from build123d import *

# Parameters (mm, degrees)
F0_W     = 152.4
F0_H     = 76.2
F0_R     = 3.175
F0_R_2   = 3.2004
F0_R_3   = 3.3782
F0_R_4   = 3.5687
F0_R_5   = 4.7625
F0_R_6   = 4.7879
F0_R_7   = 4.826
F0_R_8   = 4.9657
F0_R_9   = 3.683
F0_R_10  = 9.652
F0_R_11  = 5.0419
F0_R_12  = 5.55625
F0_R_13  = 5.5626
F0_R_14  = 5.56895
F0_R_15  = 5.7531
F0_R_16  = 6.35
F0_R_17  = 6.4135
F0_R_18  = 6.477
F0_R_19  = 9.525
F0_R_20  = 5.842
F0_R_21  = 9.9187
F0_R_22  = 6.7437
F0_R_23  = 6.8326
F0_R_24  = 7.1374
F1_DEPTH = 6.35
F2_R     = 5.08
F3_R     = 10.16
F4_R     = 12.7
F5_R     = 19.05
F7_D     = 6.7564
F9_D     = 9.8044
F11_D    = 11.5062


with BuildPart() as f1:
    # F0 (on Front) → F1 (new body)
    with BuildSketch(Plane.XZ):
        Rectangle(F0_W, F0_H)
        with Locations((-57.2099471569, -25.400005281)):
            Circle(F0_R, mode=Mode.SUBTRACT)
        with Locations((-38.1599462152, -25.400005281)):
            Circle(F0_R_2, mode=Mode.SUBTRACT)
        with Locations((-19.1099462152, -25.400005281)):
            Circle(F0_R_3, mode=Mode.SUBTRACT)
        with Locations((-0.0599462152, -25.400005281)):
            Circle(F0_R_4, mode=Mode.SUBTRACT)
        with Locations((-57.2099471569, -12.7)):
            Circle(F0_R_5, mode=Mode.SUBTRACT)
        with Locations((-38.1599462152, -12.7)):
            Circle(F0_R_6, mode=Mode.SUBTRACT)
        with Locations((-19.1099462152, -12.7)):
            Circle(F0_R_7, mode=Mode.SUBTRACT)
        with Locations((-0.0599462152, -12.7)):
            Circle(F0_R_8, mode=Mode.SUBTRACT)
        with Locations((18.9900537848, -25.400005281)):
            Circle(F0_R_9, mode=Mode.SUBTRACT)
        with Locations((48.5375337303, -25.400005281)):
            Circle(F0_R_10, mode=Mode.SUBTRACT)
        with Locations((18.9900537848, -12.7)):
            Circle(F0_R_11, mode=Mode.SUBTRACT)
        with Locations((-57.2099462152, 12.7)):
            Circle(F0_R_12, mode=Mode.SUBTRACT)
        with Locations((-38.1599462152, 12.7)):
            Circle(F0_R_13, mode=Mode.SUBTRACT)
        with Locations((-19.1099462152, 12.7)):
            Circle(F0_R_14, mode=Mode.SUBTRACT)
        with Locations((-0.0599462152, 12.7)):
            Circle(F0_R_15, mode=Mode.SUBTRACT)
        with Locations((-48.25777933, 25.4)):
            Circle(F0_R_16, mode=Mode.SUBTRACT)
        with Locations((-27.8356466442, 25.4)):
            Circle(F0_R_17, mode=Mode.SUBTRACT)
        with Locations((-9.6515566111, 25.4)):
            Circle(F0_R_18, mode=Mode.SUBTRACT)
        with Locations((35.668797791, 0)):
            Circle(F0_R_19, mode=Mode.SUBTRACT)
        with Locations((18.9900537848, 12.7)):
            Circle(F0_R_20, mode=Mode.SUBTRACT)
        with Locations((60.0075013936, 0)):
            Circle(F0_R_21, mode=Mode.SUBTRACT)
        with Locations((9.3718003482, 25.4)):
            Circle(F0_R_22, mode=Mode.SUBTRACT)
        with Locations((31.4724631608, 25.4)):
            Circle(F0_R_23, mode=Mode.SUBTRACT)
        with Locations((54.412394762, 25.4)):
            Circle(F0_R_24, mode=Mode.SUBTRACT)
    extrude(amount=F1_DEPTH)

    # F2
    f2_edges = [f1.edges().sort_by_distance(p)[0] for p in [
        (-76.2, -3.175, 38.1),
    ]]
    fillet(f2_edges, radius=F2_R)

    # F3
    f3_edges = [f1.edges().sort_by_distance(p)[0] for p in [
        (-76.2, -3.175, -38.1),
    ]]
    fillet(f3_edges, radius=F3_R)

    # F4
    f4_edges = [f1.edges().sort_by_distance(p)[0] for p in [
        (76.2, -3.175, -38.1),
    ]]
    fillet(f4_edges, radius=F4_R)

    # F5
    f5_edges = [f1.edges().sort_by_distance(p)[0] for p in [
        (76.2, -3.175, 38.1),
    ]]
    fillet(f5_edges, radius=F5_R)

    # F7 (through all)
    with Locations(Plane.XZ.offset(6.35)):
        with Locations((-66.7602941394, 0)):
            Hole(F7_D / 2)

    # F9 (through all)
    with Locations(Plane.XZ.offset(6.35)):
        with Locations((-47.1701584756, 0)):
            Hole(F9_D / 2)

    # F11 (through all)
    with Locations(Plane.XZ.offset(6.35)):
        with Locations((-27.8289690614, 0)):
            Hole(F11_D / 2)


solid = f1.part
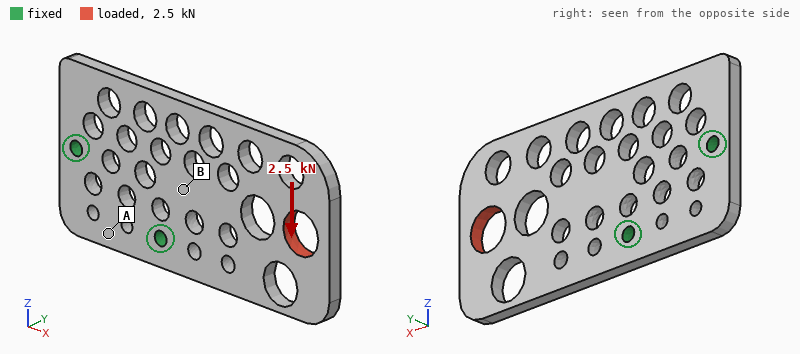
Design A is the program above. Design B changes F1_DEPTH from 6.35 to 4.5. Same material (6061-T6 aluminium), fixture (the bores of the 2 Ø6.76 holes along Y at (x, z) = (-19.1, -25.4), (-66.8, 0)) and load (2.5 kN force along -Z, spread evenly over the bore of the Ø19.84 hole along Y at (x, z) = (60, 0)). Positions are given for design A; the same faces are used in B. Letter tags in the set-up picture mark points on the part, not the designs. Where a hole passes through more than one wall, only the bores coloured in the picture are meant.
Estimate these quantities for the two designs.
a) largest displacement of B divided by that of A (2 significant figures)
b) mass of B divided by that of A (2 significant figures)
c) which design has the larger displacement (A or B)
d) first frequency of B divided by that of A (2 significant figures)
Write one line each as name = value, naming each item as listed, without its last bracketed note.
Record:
largest displacement of B divided by that of A = 1.4
mass of B divided by that of A = 0.71
which design has the larger displacement = B
first frequency of B divided by that of A = 0.72
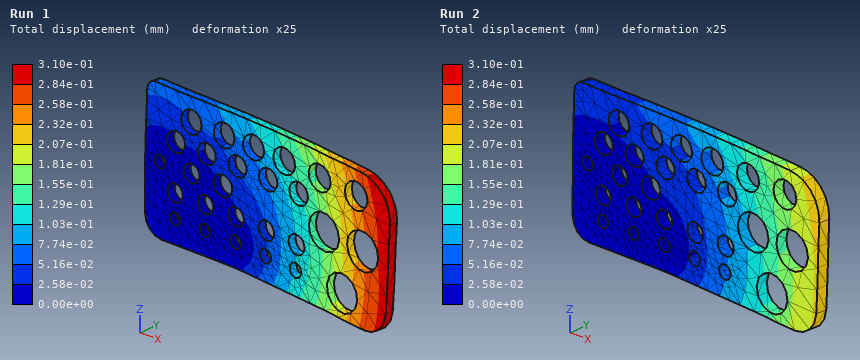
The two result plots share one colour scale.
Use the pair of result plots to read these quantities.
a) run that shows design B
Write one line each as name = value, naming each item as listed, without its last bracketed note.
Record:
run that shows design B = Run 1
